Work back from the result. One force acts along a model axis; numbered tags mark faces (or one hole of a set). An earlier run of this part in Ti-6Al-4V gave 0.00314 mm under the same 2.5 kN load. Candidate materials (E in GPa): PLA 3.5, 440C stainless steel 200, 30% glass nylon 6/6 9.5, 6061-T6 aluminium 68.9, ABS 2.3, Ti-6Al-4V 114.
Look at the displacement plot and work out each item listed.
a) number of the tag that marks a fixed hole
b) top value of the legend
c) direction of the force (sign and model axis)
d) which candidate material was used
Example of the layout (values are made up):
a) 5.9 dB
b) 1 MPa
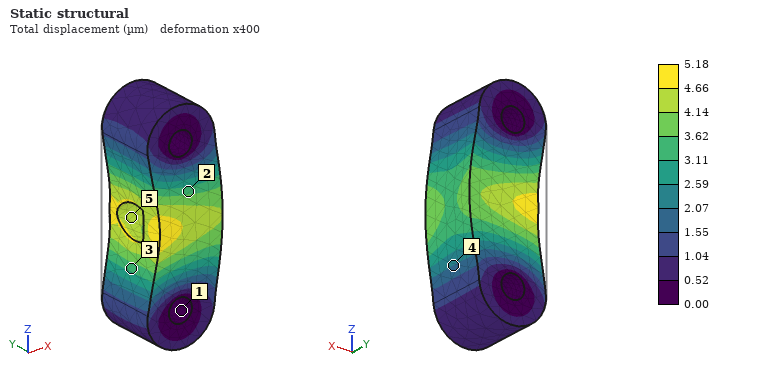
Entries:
a) 1
b) 5.18 µm
c) +X
d) 6061-T6 aluminium
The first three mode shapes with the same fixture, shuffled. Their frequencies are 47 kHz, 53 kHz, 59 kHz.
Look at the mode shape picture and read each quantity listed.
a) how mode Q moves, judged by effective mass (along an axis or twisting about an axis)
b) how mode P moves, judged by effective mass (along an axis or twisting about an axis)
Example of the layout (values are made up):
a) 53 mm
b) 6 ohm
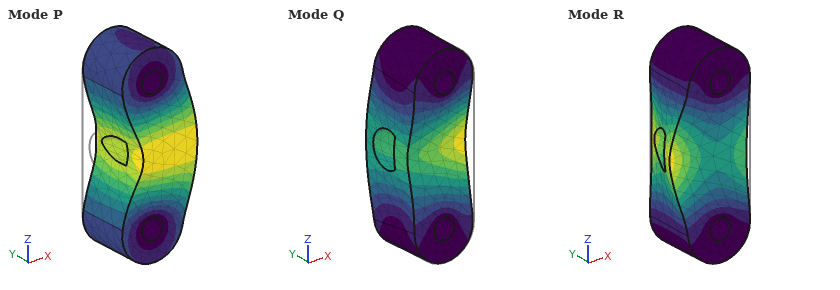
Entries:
a) along Y
b) along X
